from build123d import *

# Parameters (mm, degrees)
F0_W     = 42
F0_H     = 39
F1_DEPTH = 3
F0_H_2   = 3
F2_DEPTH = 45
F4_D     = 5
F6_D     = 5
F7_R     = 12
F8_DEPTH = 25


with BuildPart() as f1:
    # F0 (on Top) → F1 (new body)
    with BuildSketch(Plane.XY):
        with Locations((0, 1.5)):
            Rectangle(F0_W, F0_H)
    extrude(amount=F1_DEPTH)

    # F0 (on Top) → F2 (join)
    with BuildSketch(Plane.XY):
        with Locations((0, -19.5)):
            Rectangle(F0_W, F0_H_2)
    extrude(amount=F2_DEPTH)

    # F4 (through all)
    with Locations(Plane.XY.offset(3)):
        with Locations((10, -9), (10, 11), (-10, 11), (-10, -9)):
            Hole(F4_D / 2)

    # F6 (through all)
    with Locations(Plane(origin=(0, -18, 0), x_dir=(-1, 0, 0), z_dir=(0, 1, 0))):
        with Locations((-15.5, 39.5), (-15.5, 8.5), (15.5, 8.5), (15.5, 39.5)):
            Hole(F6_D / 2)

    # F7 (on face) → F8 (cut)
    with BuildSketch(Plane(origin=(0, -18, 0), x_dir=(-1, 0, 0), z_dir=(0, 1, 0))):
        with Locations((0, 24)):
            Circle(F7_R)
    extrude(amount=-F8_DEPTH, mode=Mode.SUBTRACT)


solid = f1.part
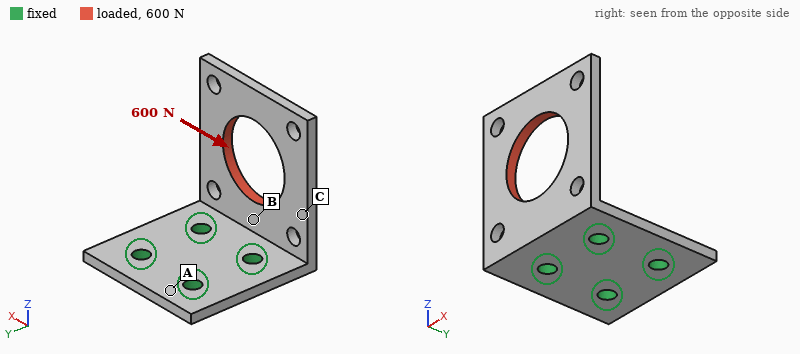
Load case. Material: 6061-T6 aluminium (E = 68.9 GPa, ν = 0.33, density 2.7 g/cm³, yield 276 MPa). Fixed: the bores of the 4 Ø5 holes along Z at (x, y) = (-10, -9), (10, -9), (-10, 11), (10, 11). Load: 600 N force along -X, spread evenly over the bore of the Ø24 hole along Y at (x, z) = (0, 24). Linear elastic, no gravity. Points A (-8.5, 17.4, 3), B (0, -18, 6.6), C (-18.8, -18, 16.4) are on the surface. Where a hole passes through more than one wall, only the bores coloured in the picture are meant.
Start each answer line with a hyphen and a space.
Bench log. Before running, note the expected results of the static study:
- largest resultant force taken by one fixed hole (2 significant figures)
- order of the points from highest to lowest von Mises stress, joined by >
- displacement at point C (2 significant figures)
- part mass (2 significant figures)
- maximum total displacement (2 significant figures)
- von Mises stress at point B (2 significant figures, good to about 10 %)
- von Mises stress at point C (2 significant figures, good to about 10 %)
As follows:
- 680 N
- B > C > A
- 0.097 mm
- 24 g
- 0.20 mm
- 62 MPa
- 30 MPa
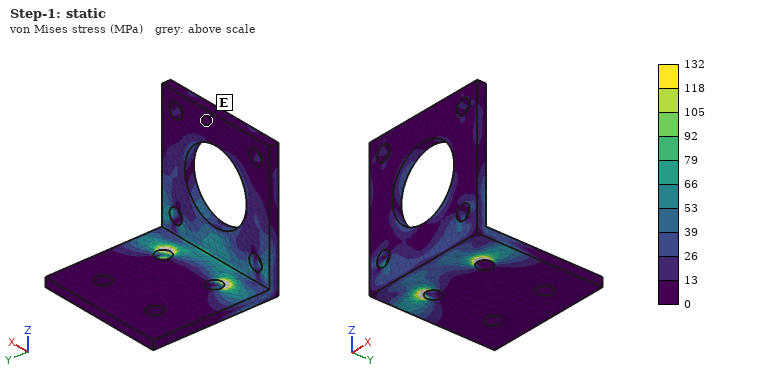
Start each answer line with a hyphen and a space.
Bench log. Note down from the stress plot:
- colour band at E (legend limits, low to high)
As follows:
- 0 to 13 MPa
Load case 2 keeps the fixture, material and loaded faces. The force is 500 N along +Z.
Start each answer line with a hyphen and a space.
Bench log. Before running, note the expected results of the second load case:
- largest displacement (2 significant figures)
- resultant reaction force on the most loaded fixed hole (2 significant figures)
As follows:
- 0.15 mm
- 270 N
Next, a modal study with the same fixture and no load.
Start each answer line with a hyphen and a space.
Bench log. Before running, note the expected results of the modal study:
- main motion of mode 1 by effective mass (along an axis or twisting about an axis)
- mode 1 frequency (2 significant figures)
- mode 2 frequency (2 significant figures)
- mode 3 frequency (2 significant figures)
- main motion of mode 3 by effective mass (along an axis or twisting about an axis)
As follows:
- along Y
- 960 Hz
- 2400 Hz
- 3500 Hz
- along X
